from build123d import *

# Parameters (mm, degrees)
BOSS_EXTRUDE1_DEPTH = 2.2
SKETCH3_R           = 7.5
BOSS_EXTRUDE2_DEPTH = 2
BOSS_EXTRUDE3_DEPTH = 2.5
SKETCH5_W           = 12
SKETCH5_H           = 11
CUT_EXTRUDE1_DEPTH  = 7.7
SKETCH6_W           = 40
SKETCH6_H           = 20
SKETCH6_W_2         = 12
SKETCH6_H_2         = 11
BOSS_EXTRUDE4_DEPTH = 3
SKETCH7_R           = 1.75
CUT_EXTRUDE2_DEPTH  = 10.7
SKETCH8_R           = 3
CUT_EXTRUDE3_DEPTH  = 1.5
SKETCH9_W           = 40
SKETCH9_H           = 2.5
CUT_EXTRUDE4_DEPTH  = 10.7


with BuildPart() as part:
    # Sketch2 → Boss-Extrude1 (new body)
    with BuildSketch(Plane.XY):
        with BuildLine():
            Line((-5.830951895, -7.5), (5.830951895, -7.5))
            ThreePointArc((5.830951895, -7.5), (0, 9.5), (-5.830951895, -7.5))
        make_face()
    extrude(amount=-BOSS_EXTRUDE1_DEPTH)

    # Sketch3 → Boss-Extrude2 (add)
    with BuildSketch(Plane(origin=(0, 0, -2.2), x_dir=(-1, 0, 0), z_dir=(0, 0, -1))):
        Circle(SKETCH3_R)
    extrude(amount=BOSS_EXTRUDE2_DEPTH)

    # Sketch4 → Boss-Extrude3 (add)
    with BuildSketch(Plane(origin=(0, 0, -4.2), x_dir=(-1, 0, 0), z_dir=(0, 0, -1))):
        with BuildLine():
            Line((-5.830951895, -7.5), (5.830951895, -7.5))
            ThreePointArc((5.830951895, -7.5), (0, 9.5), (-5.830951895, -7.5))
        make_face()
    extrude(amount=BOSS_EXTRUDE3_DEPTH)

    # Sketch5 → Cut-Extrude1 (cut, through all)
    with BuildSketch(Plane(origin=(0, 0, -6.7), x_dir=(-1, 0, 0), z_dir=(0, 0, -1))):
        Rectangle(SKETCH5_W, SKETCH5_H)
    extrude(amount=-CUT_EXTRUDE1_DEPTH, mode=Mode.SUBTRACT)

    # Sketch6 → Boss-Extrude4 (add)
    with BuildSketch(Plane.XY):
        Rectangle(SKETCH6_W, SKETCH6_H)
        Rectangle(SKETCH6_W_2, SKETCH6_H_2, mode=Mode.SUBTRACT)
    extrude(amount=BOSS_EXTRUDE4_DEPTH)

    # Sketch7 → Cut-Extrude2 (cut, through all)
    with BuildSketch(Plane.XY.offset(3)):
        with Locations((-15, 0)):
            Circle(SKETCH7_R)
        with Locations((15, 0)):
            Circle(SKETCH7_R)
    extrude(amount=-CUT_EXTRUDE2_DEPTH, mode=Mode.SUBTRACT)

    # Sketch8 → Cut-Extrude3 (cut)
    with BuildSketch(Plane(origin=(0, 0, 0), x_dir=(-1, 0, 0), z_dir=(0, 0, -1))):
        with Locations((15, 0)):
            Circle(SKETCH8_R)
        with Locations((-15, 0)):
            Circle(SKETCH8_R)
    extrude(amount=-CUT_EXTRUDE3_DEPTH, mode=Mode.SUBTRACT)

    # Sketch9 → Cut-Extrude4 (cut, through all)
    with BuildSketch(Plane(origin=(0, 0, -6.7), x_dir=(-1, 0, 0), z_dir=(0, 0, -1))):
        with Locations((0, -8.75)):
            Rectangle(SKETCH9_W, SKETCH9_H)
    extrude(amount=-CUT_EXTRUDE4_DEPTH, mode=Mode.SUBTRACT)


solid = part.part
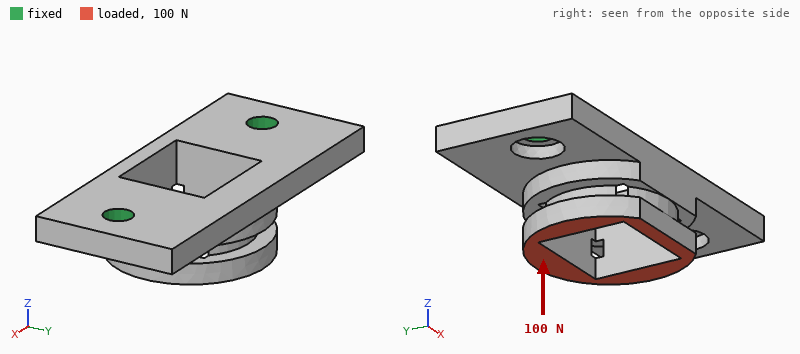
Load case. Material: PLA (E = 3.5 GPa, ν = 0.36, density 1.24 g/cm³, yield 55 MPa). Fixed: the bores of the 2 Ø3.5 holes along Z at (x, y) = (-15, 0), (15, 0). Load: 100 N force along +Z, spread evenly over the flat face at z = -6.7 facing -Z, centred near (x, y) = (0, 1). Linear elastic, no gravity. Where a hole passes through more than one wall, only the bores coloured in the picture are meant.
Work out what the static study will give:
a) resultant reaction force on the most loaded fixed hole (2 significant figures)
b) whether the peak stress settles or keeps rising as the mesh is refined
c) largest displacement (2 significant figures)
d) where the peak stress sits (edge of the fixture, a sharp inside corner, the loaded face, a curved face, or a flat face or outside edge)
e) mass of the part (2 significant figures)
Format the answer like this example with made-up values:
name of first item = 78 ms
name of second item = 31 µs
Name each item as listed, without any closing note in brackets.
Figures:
resultant reaction force on the most loaded fixed hole = 73 N
whether the peak stress settles or keeps rising as the mesh is refined = keeps rising
largest displacement = 0.12 mm
where the peak stress sits = edge of the fixture
mass of the part = 2.9 g
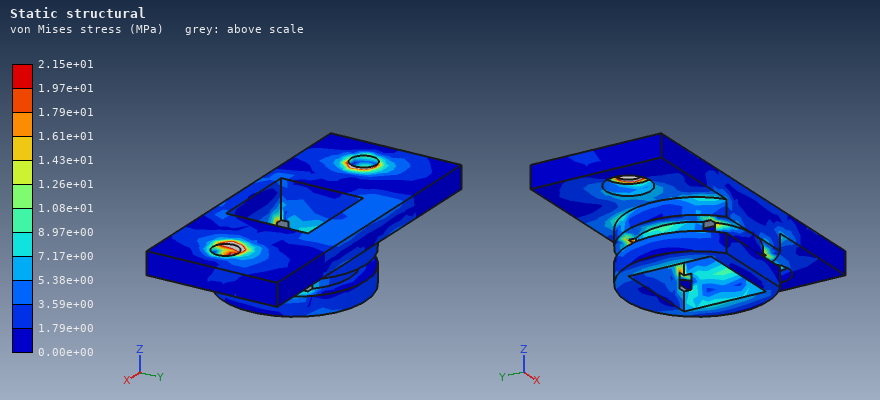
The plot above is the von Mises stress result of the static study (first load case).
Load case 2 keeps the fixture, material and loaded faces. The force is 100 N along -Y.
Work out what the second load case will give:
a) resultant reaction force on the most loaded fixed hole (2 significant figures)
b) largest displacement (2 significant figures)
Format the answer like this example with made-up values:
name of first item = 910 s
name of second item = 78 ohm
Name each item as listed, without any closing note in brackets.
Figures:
resultant reaction force on the most loaded fixed hole = 52 N
largest displacement = 0.44 mm
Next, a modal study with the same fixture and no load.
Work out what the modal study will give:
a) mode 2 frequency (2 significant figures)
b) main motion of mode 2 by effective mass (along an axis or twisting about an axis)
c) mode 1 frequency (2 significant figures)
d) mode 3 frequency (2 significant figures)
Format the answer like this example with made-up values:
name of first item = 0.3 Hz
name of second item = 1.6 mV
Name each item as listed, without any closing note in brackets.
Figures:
mode 2 frequency = 4700 Hz
main motion of mode 2 by effective mass = along Z
mode 1 frequency = 2700 Hz
mode 3 frequency = 6300 Hz
